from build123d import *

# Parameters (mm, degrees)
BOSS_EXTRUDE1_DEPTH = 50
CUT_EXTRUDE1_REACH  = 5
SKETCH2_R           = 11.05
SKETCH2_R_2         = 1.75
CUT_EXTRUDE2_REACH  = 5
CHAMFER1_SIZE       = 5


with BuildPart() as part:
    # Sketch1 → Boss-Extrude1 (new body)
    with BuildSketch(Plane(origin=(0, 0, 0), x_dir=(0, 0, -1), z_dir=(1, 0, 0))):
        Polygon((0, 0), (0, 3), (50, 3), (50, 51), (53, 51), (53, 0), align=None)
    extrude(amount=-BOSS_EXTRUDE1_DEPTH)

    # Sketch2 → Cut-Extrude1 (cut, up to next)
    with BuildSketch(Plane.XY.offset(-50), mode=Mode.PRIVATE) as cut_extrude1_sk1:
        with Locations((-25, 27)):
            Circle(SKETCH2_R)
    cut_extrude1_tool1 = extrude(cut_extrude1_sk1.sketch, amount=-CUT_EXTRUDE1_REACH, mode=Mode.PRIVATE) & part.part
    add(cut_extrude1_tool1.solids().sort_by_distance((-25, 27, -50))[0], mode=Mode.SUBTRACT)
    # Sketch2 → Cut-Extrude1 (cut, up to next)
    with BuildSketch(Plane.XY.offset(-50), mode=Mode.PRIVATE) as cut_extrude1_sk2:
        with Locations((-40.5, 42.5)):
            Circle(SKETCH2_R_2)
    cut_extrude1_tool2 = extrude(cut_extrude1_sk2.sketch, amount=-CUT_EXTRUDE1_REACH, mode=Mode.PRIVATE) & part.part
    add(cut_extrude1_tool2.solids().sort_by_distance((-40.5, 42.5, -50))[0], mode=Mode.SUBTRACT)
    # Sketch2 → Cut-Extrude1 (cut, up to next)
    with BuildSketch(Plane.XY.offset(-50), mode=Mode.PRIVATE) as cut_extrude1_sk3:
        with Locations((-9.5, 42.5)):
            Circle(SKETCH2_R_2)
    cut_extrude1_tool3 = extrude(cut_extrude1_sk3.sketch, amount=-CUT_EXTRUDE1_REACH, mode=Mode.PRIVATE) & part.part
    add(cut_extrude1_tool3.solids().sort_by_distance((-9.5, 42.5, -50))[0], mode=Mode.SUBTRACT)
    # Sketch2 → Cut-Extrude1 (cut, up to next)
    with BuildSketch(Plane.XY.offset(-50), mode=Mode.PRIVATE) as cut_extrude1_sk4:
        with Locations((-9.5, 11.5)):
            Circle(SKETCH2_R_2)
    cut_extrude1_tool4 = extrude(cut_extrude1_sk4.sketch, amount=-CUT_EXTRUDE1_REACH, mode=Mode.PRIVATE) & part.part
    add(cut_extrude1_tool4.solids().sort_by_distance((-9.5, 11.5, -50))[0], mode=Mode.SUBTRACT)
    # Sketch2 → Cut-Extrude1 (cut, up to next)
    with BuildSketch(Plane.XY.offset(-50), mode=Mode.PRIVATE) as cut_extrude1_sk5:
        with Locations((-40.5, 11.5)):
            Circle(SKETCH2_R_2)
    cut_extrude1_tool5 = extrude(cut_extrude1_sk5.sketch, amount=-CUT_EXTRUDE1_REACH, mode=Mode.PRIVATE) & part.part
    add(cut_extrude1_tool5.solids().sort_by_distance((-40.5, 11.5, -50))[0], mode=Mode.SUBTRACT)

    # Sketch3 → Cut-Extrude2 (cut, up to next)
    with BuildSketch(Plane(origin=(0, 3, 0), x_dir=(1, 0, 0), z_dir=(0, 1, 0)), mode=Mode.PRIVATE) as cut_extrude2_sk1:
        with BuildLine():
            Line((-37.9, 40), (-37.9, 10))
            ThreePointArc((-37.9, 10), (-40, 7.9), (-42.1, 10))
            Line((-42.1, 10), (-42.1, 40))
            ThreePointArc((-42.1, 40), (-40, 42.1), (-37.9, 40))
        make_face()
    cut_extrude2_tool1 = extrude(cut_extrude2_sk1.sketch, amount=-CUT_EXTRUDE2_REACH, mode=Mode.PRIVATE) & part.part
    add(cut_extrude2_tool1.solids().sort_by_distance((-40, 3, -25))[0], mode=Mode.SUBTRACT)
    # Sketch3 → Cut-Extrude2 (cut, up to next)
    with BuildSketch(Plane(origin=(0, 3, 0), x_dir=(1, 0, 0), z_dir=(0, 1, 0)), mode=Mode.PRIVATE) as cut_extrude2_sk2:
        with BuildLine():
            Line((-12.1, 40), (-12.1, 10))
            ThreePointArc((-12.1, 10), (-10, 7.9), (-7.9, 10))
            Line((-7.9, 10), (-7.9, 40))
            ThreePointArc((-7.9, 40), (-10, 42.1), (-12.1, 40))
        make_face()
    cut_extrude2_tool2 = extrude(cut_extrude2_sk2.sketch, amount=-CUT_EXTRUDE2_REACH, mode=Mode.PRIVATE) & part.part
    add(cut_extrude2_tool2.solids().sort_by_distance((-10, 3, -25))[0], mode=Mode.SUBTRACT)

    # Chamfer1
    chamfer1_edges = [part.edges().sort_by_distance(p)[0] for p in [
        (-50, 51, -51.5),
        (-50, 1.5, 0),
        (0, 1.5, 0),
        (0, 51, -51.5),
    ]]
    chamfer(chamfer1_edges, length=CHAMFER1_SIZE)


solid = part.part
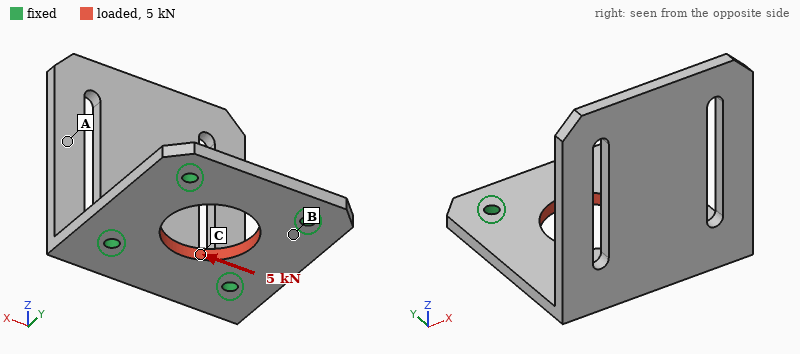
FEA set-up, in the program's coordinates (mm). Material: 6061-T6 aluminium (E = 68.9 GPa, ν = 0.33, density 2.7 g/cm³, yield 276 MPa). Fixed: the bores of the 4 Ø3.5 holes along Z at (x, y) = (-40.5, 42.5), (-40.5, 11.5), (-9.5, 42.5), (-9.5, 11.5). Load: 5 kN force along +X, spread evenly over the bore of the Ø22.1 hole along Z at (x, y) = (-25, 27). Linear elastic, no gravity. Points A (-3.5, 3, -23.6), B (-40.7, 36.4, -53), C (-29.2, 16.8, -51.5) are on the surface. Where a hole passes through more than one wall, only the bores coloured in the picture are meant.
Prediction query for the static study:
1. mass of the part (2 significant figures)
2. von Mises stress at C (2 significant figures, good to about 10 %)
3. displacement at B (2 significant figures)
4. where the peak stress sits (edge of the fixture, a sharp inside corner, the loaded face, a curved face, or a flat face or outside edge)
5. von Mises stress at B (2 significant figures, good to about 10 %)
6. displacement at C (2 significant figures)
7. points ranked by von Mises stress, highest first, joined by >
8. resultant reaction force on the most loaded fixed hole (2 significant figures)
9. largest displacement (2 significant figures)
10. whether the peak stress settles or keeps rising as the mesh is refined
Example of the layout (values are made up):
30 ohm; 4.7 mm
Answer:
35 g; 43 MPa; 5.3 µm; edge of the fixture; 26 MPa; 6.5 µm; C > B > A; 1.3 kN; 11 µm; keeps rising
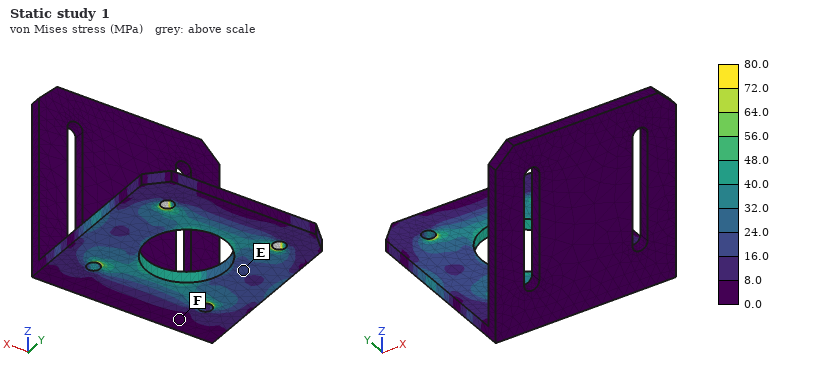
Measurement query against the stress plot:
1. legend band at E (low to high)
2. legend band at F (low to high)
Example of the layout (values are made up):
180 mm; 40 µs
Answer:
16.0 to 24.0 MPa; 0.0 to 8.0 MPa
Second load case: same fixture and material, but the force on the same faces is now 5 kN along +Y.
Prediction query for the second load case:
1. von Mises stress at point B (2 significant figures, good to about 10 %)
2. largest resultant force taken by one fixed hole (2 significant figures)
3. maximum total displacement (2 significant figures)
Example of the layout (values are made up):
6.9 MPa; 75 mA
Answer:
27 MPa; 1.3 kN; 12 µm
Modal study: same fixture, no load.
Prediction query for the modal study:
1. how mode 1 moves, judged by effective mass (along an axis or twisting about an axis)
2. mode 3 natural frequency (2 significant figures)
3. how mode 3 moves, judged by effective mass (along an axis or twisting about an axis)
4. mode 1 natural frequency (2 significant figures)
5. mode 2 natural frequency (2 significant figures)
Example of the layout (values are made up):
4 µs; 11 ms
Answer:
along Y; 3100 Hz; along X; 730 Hz; 2000 Hz
